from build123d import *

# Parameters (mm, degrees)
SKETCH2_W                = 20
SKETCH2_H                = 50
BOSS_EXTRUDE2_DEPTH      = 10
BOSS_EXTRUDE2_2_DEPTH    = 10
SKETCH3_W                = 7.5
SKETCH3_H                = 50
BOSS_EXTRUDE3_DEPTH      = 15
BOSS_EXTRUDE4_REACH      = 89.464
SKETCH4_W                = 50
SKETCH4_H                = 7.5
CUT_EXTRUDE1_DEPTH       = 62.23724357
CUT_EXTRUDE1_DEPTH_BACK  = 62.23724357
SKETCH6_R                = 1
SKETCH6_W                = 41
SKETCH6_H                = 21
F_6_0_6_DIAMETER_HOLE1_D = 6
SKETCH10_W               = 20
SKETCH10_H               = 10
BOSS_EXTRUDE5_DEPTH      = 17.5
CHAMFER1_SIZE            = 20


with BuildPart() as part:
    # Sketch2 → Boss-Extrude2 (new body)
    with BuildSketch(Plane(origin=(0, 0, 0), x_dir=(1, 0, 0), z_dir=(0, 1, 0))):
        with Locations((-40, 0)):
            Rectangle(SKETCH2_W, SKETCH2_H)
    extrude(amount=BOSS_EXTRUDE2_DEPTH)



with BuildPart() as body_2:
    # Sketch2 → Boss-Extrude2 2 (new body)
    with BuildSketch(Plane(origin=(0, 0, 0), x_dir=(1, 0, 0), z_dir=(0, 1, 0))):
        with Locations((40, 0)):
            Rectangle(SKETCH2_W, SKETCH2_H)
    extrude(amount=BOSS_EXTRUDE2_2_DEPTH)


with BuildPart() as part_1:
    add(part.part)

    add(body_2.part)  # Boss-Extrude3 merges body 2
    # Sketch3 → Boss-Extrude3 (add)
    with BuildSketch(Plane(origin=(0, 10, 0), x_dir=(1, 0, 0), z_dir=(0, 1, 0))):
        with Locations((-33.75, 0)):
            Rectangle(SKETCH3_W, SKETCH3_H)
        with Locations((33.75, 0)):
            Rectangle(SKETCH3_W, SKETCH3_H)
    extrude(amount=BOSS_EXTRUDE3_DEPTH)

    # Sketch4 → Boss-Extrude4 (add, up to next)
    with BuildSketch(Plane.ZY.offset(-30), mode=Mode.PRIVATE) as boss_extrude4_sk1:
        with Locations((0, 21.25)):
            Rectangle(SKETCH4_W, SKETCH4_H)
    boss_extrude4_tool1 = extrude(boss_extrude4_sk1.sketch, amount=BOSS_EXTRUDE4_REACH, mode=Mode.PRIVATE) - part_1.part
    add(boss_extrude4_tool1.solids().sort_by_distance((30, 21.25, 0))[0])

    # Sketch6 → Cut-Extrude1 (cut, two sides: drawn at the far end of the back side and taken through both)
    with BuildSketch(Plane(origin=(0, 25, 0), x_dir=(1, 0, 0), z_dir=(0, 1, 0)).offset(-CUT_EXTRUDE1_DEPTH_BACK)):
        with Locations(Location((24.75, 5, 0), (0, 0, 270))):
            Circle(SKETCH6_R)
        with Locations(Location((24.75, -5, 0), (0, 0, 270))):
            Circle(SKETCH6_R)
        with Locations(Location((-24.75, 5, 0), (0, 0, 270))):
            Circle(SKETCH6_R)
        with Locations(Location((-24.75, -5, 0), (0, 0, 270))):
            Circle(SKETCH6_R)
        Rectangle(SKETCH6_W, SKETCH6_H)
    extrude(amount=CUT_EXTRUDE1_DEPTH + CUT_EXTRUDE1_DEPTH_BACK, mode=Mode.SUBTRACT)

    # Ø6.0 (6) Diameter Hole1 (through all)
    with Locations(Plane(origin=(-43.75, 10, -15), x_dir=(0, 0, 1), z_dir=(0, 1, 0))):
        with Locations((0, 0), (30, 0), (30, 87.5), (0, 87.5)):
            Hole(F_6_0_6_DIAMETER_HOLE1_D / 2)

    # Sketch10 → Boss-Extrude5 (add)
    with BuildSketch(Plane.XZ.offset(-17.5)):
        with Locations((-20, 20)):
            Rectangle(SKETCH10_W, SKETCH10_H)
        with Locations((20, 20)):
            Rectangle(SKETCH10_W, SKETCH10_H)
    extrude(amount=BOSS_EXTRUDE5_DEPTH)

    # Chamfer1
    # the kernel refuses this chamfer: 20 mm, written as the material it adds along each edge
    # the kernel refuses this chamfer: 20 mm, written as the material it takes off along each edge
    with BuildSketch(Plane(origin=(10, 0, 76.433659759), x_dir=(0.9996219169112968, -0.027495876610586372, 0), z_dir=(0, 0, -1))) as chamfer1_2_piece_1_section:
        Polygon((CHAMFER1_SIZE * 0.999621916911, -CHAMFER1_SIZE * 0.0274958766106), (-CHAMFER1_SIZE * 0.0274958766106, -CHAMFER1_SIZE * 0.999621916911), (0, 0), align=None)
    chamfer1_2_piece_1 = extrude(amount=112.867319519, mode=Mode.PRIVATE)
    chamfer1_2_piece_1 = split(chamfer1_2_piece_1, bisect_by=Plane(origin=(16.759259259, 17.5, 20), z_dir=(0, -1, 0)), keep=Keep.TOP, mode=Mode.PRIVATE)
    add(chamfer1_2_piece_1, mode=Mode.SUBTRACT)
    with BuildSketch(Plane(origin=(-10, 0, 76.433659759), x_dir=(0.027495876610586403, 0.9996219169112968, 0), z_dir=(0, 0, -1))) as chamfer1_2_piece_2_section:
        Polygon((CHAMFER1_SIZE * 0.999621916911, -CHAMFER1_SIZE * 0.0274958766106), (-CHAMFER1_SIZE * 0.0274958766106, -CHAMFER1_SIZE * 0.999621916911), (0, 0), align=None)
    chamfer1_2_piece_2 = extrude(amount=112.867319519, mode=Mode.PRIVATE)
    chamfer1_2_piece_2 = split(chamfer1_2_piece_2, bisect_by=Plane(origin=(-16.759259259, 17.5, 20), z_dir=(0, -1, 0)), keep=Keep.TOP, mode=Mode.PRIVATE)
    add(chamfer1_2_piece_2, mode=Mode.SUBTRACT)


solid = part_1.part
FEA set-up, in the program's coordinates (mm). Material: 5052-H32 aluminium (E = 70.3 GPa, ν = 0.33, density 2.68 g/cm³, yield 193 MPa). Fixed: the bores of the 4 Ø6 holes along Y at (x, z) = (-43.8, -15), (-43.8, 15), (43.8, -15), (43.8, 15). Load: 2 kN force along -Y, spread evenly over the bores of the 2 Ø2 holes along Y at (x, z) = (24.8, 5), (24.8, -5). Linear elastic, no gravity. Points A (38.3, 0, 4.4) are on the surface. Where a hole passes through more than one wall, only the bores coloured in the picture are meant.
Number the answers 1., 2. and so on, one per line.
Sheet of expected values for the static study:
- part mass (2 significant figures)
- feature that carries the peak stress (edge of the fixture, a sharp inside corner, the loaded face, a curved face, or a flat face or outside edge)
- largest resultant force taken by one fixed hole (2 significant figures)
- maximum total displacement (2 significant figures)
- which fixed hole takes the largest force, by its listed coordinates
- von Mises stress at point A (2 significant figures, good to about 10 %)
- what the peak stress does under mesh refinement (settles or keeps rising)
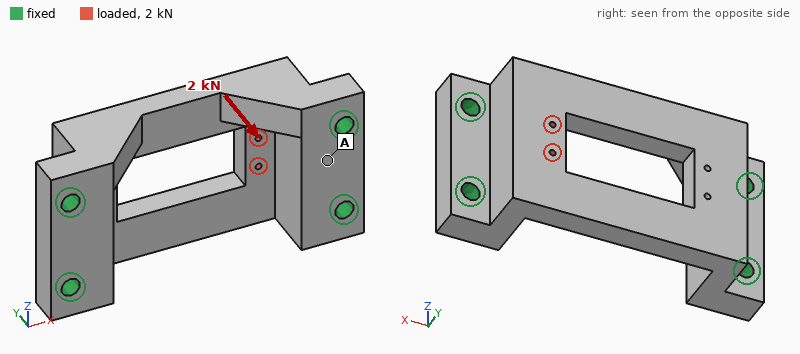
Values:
1. 130 g
2. a sharp inside corner
3. 1.0 kN
4. 27 µm
5. (43.8, -15)
6. 5.5 MPa
7. keeps rising
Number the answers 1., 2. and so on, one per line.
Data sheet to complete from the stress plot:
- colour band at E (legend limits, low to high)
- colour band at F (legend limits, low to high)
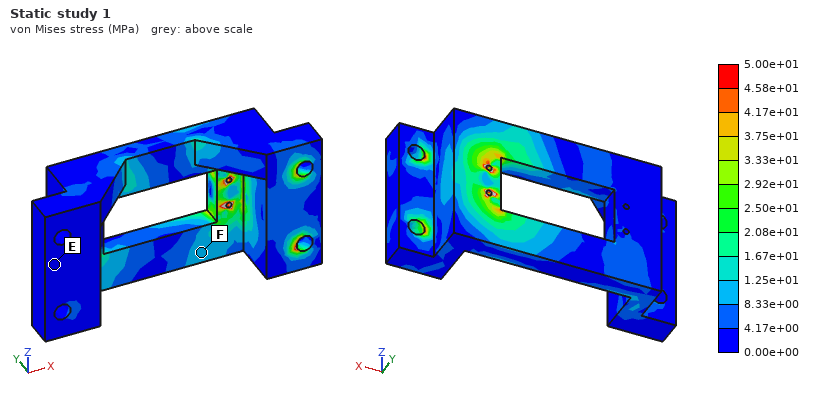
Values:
1. 0.00e+00 to 4.17e+00 MPa
2. 8.33e+00 to 1.25e+01 MPa
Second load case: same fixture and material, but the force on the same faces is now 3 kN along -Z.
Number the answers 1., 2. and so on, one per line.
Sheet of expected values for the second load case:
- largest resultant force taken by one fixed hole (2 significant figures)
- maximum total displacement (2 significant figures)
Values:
1. 2.1 kN
2. 14 µm
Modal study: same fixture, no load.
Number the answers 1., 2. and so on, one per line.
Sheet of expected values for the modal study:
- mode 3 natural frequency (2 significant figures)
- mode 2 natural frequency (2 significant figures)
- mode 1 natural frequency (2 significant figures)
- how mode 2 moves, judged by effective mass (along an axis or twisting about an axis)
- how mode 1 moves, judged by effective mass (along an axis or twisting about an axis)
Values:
1. 11 kHz
2. 9100 Hz
3. 8000 Hz
4. along X
5. along Y
